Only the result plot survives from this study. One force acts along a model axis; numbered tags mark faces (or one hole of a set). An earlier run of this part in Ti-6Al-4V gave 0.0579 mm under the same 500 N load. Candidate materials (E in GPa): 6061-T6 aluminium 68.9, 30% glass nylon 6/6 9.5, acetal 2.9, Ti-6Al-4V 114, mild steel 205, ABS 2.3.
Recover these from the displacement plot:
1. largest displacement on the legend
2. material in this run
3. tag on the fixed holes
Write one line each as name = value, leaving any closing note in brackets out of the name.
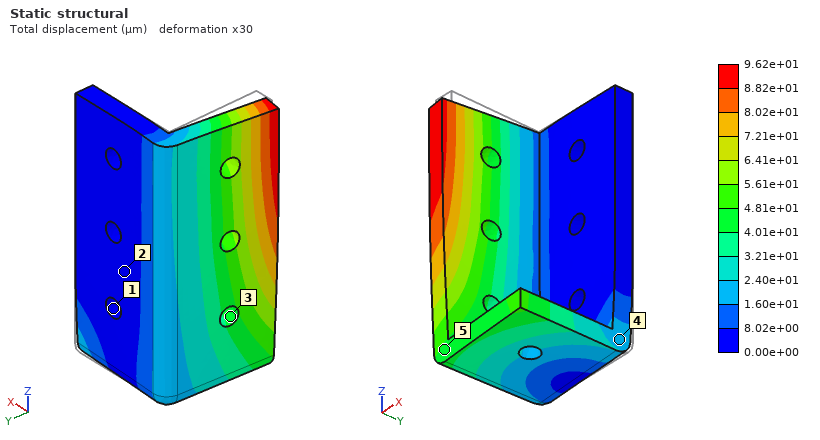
largest displacement on the legend = 9.62e+01 µm
material in this run = 6061-T6 aluminium
tag on the fixed holes = 1
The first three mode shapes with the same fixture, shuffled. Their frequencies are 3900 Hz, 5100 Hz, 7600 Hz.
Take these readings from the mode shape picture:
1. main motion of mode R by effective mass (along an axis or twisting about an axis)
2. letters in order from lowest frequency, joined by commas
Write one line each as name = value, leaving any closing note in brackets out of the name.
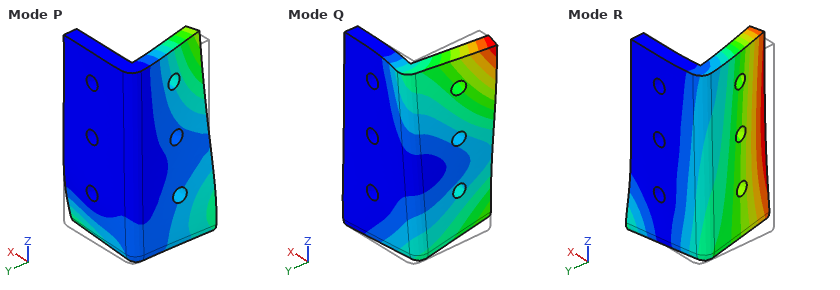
main motion of mode R by effective mass = along X
letters in order from lowest frequency, joined by commas = R, Q, P
